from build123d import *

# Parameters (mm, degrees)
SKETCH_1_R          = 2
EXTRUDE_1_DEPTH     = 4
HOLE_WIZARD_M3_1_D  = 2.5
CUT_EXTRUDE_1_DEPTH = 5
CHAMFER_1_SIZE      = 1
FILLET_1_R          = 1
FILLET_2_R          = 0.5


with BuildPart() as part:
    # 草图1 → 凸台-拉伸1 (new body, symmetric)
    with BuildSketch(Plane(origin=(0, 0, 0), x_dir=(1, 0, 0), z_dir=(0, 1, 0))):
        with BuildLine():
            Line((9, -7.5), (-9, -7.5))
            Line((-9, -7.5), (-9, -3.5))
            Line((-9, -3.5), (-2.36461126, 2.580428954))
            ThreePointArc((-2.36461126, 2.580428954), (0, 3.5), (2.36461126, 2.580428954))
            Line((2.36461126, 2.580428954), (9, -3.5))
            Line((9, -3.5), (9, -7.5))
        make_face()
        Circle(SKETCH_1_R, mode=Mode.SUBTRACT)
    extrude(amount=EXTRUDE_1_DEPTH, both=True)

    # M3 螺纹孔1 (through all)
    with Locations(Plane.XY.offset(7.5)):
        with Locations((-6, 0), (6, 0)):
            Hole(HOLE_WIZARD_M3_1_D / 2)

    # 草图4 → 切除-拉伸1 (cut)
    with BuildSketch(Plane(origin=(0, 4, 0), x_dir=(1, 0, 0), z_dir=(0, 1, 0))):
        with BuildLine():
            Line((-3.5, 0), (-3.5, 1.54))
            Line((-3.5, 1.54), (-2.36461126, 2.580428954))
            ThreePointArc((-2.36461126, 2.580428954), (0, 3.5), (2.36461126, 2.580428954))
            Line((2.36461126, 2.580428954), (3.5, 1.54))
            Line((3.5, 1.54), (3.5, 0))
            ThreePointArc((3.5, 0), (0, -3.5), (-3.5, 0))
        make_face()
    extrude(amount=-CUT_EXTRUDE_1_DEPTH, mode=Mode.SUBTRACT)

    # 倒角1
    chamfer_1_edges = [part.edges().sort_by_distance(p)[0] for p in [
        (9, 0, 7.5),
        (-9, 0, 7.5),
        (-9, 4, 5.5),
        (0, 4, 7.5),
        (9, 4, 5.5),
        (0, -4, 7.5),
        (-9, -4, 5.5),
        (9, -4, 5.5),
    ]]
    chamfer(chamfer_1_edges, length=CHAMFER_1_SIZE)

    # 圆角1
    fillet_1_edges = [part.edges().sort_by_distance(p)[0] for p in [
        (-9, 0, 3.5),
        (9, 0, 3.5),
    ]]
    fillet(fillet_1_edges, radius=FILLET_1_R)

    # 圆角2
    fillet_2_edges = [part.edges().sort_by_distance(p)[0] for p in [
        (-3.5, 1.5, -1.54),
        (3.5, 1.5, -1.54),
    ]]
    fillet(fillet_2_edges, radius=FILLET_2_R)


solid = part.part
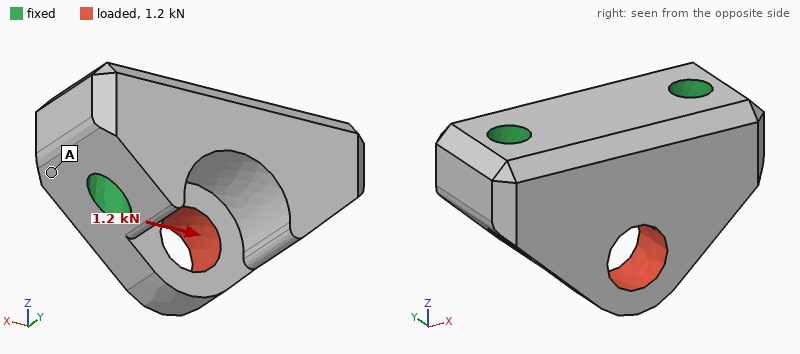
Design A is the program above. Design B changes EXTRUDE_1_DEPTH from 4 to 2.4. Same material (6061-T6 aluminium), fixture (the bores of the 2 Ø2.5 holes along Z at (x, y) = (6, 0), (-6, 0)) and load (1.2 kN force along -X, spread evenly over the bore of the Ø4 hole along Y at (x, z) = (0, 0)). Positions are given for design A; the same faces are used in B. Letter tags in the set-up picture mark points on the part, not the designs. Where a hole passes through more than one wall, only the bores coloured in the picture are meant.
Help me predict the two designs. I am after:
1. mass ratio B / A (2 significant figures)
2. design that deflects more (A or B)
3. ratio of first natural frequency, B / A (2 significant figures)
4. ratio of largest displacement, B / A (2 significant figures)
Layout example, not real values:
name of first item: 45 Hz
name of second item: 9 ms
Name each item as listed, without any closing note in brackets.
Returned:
mass ratio B / A: 0.54
design that deflects more: B
ratio of first natural frequency, B / A: 0.72
ratio of largest displacement, B / A: 1.8
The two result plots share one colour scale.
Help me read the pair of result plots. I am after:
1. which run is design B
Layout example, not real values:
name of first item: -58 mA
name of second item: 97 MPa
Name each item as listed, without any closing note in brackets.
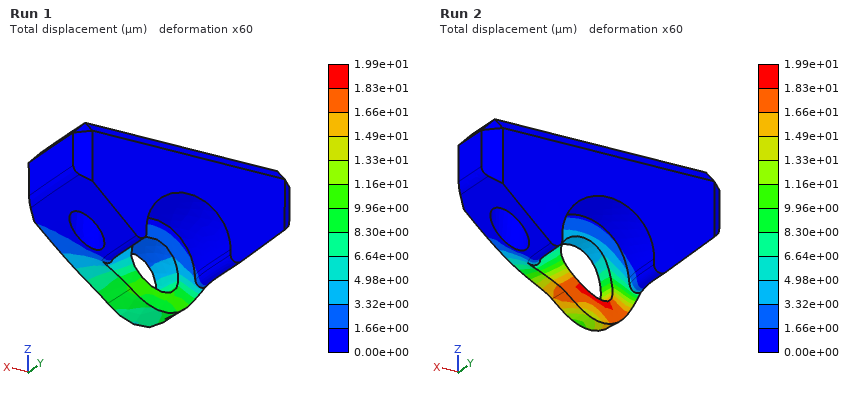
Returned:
which run is design B: Run 2
